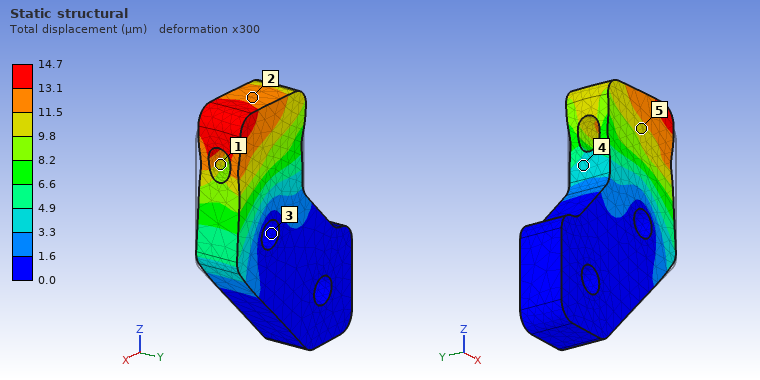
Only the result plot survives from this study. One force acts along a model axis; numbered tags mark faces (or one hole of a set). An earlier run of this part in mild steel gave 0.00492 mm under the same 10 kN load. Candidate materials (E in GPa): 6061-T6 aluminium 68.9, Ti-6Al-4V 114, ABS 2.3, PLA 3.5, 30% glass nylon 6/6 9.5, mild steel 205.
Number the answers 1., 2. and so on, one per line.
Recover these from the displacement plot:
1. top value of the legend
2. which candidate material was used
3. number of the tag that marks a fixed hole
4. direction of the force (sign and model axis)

1. 14.7 µm
2. 6061-T6 aluminium
3. 3
4. +Z
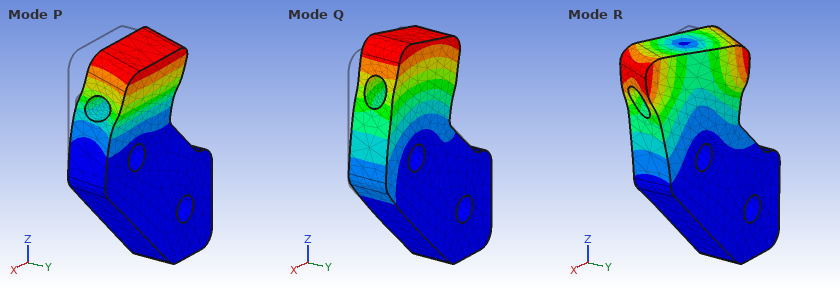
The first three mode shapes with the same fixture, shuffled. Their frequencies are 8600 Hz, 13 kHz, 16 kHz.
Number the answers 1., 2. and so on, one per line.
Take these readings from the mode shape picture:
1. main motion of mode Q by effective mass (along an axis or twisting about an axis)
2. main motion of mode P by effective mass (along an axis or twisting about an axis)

1. along X
2. along Y
